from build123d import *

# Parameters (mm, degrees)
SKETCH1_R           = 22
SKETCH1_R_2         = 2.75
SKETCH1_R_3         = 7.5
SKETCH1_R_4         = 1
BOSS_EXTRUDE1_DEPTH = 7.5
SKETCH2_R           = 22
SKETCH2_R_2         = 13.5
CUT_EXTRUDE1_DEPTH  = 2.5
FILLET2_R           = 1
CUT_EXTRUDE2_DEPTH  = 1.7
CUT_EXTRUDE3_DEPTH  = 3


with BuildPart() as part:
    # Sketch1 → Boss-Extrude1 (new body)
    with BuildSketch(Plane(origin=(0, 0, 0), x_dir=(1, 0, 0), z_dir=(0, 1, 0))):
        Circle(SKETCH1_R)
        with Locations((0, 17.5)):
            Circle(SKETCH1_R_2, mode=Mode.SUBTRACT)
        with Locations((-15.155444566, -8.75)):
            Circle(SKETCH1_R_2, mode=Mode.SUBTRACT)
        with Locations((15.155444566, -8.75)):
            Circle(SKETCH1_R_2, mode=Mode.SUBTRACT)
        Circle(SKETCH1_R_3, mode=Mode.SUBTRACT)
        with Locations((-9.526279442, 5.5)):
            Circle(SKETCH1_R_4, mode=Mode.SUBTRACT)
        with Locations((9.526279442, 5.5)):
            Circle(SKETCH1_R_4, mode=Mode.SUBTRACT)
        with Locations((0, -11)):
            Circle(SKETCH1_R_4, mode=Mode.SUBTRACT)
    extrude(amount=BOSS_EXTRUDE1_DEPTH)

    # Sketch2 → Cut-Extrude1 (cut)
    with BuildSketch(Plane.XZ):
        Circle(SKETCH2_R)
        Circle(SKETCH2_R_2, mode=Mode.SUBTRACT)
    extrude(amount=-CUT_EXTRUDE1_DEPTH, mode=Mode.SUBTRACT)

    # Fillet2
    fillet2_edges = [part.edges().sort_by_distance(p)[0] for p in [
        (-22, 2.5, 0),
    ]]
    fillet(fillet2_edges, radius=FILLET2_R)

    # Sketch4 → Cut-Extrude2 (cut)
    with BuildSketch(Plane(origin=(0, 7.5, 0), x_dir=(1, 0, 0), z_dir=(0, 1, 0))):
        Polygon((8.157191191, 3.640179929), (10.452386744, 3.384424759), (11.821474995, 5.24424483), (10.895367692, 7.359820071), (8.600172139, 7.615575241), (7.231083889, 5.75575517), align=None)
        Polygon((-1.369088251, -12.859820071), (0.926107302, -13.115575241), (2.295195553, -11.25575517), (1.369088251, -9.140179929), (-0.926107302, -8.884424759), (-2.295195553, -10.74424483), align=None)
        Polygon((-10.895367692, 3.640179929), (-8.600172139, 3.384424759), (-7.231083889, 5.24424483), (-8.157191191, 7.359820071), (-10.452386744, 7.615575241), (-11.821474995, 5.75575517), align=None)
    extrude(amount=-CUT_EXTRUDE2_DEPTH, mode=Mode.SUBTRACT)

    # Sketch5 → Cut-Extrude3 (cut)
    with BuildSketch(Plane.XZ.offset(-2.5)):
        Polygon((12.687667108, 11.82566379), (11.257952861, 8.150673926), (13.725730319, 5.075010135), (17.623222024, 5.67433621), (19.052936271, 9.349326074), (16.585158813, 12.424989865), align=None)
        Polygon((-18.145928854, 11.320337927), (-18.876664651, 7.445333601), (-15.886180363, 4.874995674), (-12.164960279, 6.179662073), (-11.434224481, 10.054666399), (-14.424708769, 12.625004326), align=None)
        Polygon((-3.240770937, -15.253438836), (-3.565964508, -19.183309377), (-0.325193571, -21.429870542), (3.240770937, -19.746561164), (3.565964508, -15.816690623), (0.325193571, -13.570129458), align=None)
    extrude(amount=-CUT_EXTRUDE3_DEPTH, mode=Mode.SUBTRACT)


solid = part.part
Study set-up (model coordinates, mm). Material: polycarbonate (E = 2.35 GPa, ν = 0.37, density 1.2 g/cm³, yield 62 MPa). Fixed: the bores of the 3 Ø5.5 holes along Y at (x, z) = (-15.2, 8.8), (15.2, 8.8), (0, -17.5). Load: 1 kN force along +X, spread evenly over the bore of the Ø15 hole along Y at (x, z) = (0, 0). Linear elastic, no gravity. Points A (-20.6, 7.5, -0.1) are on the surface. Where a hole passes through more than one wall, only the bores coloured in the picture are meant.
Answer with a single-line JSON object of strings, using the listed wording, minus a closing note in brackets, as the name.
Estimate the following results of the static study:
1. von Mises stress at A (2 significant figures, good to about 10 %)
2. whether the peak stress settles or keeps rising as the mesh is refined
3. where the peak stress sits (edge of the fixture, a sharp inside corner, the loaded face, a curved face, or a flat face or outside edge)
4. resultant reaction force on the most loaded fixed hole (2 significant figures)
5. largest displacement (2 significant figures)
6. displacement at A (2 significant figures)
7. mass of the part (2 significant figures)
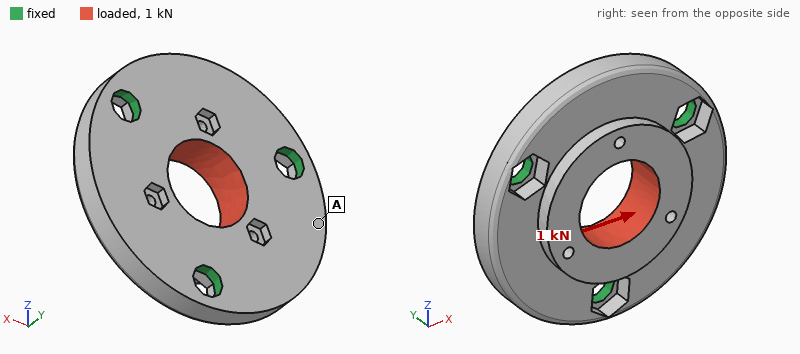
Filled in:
{"von Mises stress at A": "2.8 MPa", "whether the peak stress settles or keeps rising as the mesh is refined": "keeps rising", "where the peak stress sits": "edge of the fixture", "resultant reaction force on the most loaded fixed hole": "350 N", "largest displacement": "91 µm", "displacement at A": "51 µm", "mass of the part": "8.5 g"}
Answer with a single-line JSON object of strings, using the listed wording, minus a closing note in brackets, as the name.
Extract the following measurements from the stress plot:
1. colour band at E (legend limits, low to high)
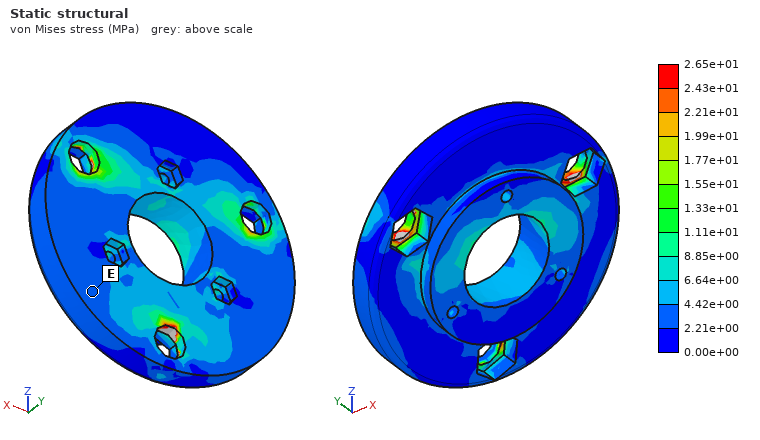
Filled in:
{"colour band at E": "2.21e+00 to 4.42e+00 MPa"}
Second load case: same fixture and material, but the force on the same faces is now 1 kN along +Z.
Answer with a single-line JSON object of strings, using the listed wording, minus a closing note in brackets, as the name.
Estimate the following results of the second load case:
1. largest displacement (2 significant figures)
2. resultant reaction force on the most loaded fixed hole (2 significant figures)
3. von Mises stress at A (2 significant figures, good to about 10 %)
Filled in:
{"largest displacement": "0.11 mm", "resultant reaction force on the most loaded fixed hole": "360 N", "von Mises stress at A": "3.3 MPa"}
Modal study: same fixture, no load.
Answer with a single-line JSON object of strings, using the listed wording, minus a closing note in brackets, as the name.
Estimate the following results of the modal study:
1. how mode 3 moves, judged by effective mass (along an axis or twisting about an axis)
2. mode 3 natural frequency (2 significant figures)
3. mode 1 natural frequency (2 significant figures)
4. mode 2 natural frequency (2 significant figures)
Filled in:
{"how mode 3 moves, judged by effective mass": "along Y", "mode 3 natural frequency": "5400 Hz", "mode 1 natural frequency": "4200 Hz", "mode 2 natural frequency": "4200 Hz"}
